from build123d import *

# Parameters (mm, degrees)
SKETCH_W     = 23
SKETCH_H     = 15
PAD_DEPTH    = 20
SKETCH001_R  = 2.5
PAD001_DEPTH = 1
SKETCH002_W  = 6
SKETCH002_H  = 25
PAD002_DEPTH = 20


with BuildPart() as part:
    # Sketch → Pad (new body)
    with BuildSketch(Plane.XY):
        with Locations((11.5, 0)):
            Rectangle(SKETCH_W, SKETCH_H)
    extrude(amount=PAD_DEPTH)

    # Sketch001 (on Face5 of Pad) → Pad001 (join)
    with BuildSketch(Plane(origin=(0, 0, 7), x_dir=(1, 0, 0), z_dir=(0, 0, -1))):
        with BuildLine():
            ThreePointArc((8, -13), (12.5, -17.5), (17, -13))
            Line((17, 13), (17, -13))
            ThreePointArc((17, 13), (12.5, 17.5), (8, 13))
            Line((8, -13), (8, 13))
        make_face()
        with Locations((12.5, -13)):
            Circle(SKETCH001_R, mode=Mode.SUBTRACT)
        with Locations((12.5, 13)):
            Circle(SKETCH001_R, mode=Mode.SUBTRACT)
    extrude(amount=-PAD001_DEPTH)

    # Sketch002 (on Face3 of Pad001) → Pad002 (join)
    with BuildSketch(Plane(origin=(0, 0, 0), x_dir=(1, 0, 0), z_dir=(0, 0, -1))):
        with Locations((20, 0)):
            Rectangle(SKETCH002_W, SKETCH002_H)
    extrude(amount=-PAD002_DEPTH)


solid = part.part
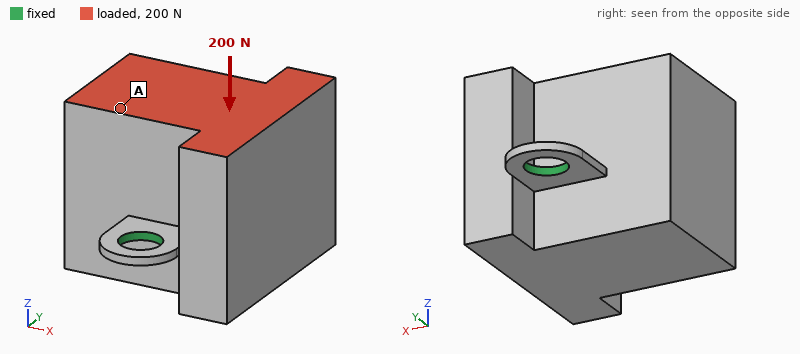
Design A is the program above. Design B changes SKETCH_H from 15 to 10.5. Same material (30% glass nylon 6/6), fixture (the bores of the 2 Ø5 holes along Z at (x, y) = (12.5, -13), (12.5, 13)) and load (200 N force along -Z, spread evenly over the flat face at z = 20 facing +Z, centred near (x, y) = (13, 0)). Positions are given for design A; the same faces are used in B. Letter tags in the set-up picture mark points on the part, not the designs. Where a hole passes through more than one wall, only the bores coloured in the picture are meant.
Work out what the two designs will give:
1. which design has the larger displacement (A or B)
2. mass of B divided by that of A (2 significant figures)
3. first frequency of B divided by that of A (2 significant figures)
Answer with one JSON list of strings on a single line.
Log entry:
["B", "0.82", "0.80"]
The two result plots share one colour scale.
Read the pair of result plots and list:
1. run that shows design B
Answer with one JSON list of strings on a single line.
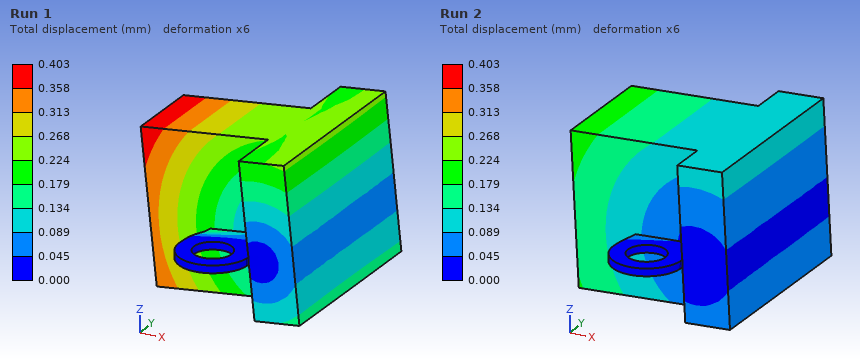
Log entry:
["Run 1"]
